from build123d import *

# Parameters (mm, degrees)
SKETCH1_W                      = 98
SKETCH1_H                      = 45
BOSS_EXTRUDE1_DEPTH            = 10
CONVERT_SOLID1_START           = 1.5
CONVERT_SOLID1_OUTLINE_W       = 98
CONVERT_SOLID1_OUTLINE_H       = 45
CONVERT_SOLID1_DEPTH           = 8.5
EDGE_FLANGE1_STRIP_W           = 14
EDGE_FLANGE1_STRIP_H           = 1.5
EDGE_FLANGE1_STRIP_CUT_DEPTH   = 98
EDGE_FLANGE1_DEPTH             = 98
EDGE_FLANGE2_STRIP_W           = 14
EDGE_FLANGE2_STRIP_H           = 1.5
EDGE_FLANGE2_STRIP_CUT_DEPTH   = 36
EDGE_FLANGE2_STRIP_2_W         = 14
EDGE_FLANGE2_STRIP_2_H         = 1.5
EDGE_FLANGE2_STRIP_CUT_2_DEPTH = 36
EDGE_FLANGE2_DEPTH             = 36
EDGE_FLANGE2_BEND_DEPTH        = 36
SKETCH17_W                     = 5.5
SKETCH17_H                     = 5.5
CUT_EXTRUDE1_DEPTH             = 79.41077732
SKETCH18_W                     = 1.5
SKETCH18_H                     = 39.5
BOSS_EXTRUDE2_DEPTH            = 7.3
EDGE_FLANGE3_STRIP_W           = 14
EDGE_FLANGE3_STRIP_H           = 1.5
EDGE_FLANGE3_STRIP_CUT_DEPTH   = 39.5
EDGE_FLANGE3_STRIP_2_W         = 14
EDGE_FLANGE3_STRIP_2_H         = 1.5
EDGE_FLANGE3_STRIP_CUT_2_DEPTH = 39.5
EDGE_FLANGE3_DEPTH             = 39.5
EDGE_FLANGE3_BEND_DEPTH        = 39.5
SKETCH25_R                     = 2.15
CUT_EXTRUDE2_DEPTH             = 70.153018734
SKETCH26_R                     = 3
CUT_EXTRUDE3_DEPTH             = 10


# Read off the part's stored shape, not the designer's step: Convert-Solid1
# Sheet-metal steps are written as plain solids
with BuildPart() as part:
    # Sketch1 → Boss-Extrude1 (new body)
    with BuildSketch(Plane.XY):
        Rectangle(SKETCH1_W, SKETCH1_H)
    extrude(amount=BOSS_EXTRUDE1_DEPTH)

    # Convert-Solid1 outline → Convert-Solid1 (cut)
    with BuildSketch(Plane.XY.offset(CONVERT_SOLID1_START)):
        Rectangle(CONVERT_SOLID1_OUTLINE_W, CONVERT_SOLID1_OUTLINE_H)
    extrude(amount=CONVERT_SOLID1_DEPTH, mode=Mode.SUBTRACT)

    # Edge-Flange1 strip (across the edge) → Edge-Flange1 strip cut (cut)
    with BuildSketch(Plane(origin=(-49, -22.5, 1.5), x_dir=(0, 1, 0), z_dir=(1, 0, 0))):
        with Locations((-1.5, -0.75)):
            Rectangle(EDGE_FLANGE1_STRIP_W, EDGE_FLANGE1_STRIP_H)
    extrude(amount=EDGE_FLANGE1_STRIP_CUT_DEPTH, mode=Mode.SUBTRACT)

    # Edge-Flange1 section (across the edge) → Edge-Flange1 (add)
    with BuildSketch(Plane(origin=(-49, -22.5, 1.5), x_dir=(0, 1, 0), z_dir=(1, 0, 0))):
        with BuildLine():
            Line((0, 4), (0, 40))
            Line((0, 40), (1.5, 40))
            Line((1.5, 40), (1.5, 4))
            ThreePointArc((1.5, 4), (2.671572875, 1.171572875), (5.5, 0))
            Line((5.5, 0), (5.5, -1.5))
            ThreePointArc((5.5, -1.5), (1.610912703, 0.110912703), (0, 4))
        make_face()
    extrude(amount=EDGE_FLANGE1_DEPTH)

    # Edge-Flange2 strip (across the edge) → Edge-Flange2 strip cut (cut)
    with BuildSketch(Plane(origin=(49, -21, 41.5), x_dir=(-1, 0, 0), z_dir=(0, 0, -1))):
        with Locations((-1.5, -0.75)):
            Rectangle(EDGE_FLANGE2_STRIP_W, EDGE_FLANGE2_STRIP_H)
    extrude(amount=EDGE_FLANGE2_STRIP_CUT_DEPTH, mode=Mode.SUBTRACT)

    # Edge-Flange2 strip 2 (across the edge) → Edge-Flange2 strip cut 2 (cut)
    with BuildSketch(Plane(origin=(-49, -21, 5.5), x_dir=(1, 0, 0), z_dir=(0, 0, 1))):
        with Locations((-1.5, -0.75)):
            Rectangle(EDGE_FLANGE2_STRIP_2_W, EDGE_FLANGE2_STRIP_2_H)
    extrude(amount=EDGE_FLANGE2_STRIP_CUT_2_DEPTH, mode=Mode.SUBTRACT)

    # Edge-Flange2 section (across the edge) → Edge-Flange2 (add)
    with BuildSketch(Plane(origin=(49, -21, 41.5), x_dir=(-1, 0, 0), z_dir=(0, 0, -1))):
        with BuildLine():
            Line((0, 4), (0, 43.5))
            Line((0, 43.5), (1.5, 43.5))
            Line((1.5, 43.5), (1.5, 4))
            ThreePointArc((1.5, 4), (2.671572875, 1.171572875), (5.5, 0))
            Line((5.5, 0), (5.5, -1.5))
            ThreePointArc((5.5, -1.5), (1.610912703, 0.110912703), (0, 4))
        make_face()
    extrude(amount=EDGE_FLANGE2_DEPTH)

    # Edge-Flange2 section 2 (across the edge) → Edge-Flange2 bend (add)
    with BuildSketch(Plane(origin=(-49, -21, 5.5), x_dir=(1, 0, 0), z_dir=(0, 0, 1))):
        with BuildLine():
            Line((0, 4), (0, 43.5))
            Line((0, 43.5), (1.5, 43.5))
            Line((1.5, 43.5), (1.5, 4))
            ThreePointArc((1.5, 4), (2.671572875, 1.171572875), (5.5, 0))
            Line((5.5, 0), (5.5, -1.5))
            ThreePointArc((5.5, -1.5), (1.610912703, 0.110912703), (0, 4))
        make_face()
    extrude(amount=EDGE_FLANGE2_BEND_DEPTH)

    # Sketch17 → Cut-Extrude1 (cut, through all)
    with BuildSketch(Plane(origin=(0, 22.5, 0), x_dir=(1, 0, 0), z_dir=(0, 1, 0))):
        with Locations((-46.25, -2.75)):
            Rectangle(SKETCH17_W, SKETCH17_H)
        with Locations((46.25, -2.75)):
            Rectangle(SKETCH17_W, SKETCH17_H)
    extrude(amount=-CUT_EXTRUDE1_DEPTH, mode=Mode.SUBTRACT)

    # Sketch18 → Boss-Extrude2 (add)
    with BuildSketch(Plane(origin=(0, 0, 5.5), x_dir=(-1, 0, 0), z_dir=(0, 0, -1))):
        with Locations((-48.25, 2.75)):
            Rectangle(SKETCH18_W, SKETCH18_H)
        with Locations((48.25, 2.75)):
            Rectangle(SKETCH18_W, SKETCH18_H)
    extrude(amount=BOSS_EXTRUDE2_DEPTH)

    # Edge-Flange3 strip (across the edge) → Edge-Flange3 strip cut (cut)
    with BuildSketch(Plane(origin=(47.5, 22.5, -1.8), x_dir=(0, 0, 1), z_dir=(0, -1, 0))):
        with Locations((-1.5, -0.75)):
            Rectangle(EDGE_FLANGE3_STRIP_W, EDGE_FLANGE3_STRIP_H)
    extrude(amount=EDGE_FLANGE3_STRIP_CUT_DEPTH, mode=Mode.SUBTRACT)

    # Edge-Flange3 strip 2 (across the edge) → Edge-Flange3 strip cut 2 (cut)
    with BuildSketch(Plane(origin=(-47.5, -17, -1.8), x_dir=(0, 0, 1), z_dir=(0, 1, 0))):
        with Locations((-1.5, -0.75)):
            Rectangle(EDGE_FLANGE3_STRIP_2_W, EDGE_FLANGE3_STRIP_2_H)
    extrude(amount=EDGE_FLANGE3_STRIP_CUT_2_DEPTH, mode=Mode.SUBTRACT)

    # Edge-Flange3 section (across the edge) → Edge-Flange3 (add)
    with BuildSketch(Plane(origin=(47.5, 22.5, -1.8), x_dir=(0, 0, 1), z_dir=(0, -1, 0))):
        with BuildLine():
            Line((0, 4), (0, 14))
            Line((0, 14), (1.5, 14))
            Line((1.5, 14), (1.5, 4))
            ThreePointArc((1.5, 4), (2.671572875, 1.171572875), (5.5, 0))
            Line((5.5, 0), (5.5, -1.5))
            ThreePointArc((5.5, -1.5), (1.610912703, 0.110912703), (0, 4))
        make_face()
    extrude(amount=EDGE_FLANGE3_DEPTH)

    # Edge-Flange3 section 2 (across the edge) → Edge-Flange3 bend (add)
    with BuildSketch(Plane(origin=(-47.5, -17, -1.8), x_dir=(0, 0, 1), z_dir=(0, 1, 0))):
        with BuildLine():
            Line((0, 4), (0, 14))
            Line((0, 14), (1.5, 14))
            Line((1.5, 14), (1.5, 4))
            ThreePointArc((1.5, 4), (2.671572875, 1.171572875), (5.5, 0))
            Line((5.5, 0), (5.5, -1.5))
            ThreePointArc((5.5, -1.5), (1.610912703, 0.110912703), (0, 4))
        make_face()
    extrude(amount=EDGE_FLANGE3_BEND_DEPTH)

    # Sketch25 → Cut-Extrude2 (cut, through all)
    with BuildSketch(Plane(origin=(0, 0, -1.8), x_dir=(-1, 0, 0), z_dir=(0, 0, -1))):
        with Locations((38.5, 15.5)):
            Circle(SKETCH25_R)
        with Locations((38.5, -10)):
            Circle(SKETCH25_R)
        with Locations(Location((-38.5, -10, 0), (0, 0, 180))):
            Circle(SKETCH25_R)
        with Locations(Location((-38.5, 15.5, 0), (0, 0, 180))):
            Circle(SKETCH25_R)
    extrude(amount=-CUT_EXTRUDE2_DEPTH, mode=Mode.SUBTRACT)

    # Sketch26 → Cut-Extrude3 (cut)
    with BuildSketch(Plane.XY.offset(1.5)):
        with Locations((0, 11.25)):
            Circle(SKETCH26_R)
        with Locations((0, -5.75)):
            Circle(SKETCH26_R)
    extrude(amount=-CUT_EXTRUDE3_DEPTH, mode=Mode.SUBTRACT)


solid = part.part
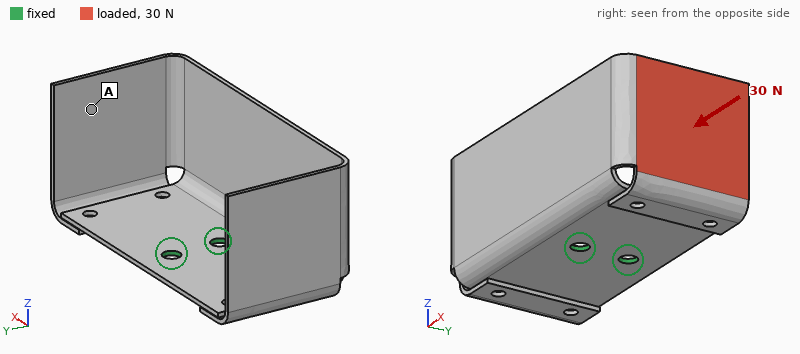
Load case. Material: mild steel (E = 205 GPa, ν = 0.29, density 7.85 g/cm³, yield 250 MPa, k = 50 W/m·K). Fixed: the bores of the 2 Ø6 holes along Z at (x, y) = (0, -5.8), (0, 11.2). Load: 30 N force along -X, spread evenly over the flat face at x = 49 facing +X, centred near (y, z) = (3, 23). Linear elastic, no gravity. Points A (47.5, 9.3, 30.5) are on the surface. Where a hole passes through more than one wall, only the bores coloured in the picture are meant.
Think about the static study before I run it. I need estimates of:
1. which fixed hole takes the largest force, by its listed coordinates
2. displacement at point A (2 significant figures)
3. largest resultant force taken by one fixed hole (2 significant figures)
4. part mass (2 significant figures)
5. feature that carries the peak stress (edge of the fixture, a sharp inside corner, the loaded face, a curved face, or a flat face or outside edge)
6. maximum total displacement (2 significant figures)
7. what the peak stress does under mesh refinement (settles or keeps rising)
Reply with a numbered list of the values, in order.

1. (0, 11.2)
2. 0.33 mm
3. 18 N
4. 140 g
5. a sharp inside corner
6. 0.49 mm
7. keeps rising
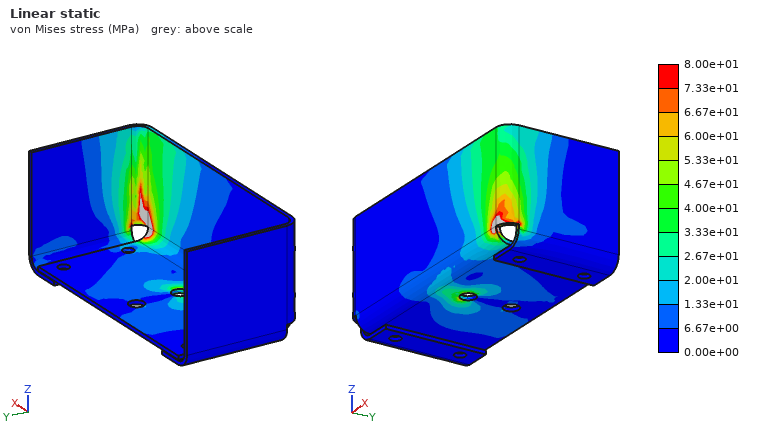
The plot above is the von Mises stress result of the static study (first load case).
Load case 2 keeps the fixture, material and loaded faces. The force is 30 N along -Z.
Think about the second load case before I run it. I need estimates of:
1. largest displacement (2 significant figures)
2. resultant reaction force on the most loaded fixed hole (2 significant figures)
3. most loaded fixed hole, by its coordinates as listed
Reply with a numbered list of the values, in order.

1. 0.49 mm
2. 20 N
3. (0, -5.8)
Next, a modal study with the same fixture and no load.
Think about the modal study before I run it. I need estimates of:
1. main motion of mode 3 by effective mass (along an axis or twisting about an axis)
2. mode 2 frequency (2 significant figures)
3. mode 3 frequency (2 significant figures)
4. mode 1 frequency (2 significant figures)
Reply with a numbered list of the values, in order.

1. along X
2. 240 Hz
3. 270 Hz
4. 230 Hz
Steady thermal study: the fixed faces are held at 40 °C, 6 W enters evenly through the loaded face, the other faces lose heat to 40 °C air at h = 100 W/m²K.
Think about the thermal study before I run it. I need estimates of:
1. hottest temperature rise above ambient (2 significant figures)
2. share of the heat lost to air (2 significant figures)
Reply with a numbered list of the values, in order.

1. 22 K
2. 99 %
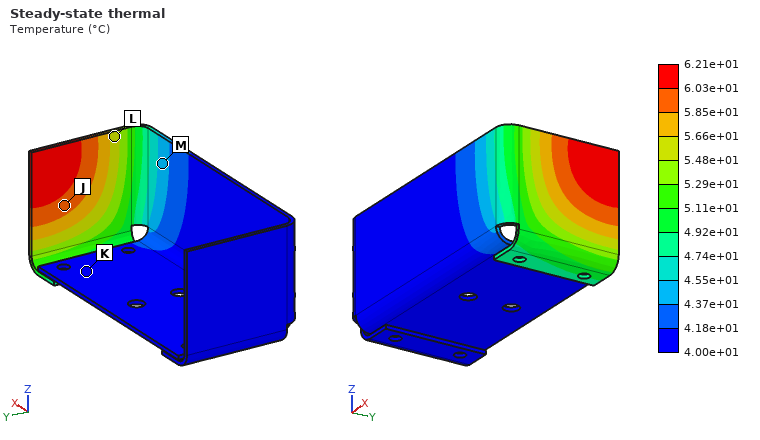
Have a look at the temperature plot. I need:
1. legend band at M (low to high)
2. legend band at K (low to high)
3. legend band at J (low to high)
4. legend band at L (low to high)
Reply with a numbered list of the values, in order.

1. 4.37e+01 to 4.55e+01 °C
2. 4.00e+01 to 4.18e+01 °C
3. 5.85e+01 to 6.03e+01 °C
4. 5.48e+01 to 5.66e+01 °C
